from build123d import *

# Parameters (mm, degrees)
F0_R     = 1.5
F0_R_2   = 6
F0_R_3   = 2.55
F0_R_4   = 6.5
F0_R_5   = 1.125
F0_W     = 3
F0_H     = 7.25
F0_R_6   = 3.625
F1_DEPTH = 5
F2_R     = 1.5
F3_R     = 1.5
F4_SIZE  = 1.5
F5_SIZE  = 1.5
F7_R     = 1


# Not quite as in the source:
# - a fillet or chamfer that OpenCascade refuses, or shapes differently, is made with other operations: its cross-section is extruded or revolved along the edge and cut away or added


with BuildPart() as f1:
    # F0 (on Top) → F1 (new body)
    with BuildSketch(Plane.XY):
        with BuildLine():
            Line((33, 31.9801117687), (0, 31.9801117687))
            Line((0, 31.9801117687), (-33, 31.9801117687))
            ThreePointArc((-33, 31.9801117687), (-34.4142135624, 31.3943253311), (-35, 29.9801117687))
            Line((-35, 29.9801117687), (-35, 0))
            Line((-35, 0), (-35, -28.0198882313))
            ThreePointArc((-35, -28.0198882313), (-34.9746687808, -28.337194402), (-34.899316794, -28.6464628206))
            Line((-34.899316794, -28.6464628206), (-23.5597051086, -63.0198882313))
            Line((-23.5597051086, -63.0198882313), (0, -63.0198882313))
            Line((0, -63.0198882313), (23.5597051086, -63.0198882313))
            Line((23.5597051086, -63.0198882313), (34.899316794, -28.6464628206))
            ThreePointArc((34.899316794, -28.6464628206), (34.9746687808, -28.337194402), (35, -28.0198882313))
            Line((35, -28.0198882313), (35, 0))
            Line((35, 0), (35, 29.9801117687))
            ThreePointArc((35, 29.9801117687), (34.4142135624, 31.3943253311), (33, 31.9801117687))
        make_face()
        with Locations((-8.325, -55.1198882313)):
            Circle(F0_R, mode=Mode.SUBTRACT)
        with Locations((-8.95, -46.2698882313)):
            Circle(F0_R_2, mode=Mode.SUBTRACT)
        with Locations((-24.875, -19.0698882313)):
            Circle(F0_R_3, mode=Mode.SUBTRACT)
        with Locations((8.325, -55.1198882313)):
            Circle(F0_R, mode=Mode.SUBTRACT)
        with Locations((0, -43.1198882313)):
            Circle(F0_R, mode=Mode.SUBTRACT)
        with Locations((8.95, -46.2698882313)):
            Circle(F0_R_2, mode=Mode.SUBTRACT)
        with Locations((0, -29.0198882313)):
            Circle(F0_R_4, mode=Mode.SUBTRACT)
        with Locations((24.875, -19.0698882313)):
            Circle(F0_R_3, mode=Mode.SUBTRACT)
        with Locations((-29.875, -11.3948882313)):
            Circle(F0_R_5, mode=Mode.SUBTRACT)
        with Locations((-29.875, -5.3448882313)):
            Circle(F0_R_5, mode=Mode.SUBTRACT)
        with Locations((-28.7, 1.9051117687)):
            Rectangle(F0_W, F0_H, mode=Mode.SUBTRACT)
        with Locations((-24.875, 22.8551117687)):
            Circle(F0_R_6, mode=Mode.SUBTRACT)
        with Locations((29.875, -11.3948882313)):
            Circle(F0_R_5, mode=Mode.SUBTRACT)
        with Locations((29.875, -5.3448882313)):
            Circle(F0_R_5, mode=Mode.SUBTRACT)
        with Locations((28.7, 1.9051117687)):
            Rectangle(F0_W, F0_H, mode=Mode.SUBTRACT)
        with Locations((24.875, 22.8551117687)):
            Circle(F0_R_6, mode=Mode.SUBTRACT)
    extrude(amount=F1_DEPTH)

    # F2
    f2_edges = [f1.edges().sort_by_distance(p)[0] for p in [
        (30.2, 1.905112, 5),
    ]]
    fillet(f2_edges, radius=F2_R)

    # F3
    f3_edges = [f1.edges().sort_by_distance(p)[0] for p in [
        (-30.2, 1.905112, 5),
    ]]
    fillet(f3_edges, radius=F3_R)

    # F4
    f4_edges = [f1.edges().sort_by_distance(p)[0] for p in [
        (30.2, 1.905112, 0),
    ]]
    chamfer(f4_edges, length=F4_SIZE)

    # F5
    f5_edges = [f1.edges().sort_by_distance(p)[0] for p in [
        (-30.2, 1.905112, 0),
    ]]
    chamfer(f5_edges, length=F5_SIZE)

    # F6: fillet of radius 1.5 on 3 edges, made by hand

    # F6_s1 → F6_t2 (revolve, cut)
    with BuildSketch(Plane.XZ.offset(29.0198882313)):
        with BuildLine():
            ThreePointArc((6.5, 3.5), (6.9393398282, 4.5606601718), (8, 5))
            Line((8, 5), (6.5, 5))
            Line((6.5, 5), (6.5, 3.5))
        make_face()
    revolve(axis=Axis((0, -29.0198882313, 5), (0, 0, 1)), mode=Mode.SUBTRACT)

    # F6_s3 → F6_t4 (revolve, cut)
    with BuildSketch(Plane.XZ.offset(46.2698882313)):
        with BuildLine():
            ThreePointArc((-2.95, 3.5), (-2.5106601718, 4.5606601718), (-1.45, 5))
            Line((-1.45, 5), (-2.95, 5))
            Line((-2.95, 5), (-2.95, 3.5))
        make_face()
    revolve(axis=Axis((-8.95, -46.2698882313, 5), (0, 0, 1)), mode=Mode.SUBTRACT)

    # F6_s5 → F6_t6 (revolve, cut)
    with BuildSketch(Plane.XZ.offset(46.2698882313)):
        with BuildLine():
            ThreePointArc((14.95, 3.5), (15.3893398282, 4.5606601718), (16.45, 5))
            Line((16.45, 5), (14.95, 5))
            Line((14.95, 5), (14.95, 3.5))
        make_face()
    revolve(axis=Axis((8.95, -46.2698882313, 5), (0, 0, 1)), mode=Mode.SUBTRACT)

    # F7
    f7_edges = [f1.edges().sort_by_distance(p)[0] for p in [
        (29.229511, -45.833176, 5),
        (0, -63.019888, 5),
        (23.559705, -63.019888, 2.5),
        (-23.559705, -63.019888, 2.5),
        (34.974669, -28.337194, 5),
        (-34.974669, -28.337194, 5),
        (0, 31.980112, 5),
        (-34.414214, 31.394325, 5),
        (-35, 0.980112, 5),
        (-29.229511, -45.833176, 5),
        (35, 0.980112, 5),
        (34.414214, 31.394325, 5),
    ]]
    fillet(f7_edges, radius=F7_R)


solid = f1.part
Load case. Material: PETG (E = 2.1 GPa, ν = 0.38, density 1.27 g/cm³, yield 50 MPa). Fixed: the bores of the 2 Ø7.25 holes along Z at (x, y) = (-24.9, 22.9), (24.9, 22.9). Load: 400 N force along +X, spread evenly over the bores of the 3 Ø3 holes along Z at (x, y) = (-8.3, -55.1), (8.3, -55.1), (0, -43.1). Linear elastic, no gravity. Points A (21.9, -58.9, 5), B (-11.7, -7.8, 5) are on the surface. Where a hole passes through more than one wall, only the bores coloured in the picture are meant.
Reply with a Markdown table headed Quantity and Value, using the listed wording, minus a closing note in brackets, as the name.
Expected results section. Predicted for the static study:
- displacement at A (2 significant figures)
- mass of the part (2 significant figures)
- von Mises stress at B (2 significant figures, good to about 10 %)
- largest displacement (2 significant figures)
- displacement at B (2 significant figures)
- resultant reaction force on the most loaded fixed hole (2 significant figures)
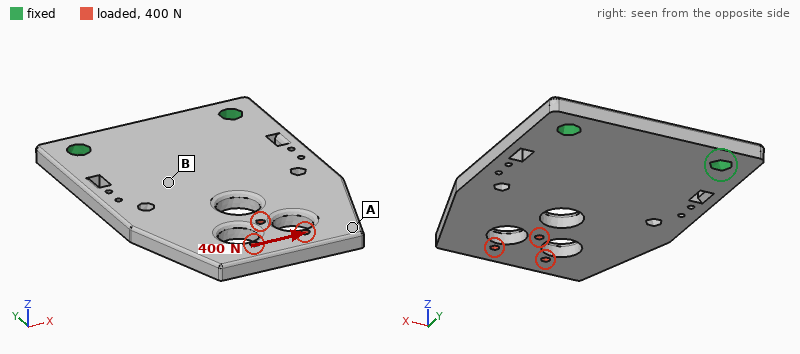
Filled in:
| Quantity | Value |
|---|---|
| displacement at A | 0.45 mm |
| mass of the part | 36 g |
| von Mises stress at B | 2.9 MPa |
| largest displacement | 0.47 mm |
| displacement at B | 0.10 mm |
| resultant reaction force on the most loaded fixed hole | 590 N |
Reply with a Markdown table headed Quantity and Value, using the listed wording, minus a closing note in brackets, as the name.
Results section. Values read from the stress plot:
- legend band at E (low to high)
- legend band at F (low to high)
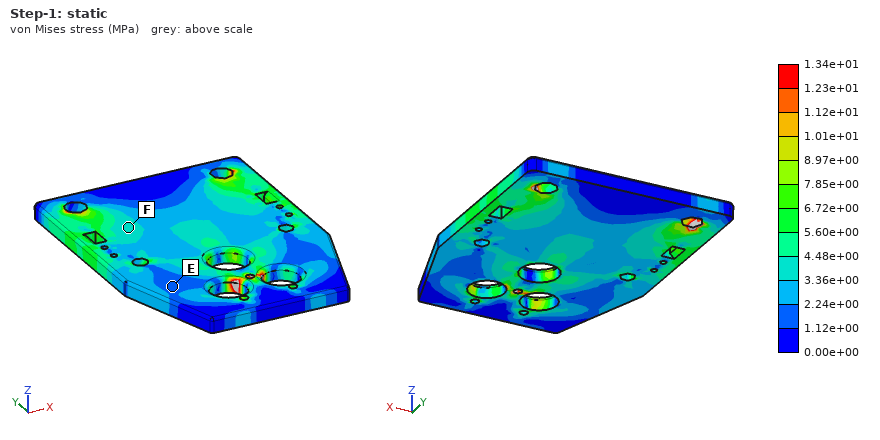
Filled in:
| Quantity | Value |
|---|---|
| legend band at E | 1.12e+00 to 2.24e+00 MPa |
| legend band at F | 3.36e+00 to 4.48e+00 MPa |
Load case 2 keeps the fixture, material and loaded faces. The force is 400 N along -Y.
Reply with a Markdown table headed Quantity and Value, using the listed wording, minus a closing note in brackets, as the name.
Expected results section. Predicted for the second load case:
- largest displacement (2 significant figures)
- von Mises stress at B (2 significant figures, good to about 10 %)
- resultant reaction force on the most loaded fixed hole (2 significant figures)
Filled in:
| Quantity | Value |
|---|---|
| largest displacement | 0.11 mm |
| von Mises stress at B | 1.3 MPa |
| resultant reaction force on the most loaded fixed hole | 200 N |
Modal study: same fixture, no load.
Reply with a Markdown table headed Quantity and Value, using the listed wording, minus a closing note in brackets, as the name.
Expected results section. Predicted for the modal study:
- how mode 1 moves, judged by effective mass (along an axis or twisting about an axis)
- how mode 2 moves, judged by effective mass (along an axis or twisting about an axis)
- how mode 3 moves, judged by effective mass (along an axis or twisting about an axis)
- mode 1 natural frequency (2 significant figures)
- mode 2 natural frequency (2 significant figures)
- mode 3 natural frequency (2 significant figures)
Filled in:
| Quantity | Value |
|---|---|
| how mode 1 moves, judged by effective mass | along Z |
| how mode 2 moves, judged by effective mass | twisting about Y |
| how mode 3 moves, judged by effective mass | along Z |
| mode 1 natural frequency | 160 Hz |
| mode 2 natural frequency | 480 Hz |
| mode 3 natural frequency | 860 Hz |
